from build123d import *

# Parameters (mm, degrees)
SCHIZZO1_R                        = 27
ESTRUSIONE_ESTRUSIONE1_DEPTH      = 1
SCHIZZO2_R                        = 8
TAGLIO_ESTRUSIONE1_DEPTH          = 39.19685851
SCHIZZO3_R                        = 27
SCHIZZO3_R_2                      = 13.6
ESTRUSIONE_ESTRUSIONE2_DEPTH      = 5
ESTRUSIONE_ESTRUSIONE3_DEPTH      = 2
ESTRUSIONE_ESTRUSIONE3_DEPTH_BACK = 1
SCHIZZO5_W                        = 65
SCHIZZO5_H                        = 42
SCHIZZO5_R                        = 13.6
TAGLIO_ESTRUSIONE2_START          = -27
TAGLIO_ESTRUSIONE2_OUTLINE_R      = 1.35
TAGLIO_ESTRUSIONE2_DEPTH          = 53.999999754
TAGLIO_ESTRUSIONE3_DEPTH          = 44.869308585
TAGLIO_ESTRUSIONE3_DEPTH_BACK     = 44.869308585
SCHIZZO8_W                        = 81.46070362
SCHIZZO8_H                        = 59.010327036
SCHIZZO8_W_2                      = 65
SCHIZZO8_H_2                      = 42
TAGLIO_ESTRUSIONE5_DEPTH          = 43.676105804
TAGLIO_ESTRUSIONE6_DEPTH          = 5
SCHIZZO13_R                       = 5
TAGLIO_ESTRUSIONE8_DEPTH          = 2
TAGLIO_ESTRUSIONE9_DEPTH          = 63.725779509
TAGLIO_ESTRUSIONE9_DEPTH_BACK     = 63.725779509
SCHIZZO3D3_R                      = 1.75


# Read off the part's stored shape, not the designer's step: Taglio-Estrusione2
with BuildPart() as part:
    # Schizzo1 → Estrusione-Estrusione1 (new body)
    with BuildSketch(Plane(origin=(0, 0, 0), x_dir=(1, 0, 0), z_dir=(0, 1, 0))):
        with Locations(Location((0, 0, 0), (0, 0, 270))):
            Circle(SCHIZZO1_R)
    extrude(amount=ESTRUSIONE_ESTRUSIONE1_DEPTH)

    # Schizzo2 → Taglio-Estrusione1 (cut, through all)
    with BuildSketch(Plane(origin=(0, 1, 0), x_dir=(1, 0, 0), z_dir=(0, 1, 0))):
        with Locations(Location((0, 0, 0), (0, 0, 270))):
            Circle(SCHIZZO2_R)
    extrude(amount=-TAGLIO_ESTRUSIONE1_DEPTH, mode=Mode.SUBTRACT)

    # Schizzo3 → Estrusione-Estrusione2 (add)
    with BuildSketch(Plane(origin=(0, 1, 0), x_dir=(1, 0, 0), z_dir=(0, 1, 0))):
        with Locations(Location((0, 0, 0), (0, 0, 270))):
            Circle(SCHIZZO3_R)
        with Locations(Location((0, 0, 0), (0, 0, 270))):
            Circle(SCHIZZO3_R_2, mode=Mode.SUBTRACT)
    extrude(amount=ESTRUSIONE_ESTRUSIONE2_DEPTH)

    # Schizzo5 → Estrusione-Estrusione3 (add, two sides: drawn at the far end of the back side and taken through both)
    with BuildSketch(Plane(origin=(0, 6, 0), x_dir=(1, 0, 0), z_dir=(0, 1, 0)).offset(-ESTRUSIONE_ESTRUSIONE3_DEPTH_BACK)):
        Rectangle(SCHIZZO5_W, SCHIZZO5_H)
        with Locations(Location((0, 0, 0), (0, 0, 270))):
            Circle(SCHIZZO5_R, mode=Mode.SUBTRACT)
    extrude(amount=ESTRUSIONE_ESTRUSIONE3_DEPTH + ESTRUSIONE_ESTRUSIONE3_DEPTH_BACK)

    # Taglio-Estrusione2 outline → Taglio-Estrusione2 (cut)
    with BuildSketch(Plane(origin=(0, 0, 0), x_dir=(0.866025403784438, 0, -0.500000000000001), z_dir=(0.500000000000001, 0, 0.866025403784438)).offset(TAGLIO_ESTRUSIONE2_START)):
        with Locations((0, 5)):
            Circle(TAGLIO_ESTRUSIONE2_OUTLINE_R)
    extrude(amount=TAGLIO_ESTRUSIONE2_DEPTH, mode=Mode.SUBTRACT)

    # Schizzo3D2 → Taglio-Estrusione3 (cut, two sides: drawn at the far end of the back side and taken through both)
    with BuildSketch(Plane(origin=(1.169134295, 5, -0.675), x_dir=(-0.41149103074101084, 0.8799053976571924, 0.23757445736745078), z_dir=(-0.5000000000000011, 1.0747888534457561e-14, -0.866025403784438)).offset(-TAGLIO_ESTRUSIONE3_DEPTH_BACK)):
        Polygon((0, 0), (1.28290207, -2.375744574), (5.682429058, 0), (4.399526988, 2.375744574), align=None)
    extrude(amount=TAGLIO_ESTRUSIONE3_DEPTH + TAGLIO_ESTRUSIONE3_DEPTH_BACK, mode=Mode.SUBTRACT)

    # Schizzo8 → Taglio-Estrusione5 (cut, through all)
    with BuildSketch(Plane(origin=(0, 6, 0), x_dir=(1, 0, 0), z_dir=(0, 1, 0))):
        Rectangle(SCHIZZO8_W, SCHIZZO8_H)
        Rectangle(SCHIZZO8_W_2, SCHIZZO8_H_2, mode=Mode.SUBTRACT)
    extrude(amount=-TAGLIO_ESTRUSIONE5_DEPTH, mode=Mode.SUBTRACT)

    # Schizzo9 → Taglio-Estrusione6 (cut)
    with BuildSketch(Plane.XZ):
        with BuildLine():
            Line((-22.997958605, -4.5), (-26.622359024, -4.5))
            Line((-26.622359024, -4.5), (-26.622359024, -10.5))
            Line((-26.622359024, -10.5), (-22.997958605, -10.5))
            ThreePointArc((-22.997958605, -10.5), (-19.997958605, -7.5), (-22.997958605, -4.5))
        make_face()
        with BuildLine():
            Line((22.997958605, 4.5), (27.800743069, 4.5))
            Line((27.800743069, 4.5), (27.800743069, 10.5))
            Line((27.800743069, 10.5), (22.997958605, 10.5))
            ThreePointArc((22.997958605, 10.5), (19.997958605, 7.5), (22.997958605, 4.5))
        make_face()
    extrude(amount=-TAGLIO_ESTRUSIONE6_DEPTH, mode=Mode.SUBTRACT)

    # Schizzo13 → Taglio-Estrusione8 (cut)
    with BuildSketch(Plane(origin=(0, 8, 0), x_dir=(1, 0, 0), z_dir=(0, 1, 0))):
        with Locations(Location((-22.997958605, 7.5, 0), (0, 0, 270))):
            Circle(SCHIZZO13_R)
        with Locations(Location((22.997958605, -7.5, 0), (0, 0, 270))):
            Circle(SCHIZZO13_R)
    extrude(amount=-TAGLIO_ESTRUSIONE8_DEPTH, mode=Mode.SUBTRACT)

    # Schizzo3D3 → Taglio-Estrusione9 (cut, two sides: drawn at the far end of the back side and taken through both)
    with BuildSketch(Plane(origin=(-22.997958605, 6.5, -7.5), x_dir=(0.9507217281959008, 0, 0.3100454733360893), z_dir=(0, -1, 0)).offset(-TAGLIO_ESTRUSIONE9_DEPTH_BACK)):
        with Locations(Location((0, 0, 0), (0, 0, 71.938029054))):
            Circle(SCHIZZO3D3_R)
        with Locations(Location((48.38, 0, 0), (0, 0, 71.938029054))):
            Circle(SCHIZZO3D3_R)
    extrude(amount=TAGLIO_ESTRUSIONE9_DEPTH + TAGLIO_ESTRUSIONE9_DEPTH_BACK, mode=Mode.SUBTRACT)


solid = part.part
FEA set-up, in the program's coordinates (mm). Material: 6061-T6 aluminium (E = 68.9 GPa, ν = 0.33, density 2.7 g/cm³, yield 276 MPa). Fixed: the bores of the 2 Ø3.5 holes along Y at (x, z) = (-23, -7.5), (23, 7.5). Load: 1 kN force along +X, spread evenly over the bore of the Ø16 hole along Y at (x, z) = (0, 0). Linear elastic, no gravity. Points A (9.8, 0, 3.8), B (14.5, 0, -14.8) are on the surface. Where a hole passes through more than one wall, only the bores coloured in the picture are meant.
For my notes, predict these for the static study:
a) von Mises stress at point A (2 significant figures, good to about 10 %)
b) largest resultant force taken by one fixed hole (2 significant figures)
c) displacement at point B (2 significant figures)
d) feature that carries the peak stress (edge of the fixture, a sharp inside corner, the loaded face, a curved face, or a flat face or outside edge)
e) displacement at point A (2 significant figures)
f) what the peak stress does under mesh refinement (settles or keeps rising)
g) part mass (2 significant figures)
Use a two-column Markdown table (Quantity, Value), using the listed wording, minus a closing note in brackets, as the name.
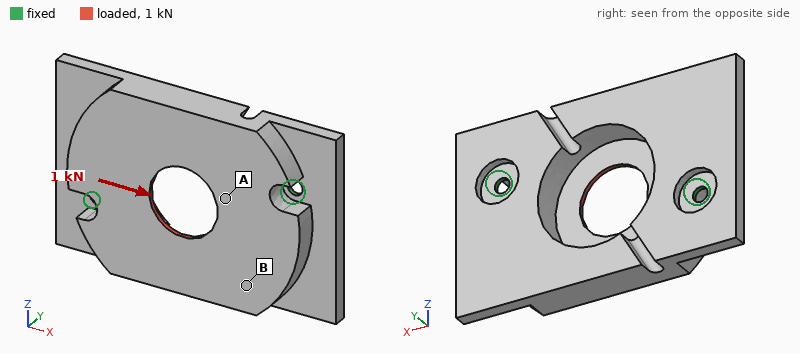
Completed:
| Quantity | Value |
|---|---|
| von Mises stress at point A | 22 MPa |
| largest resultant force taken by one fixed hole | 510 N |
| displacement at point B | 56 µm |
| feature that carries the peak stress | edge of the fixture |
| displacement at point A | 20 µm |
| what the peak stress does under mesh refinement | keeps rising |
| part mass | 35 g |
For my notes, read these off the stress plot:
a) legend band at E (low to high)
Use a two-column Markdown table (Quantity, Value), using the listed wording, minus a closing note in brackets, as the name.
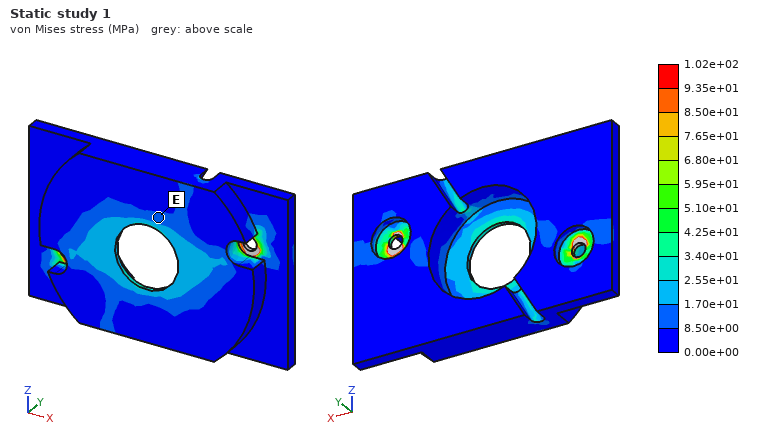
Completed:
| Quantity | Value |
|---|---|
| legend band at E | 8.50e+00 to 1.70e+01 MPa |
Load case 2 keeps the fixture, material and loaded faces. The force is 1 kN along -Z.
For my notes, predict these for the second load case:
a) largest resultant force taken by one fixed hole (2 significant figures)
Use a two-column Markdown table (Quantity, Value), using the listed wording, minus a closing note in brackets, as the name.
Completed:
| Quantity | Value |
|---|---|
| largest resultant force taken by one fixed hole | 500 N |
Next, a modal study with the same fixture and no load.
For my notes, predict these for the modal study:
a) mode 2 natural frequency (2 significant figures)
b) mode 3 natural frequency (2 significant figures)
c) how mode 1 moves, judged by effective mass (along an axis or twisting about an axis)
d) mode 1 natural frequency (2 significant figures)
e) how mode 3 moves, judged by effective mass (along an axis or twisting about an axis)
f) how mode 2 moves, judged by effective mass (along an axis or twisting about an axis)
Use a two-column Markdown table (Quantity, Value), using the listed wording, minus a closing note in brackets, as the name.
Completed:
| Quantity | Value |
|---|---|
| mode 2 natural frequency | 5000 Hz |
| mode 3 natural frequency | 6700 Hz |
| how mode 1 moves, judged by effective mass | twisting about X |
| mode 1 natural frequency | 1400 Hz |
| how mode 3 moves, judged by effective mass | along Y |
| how mode 2 moves, judged by effective mass | along Y |
